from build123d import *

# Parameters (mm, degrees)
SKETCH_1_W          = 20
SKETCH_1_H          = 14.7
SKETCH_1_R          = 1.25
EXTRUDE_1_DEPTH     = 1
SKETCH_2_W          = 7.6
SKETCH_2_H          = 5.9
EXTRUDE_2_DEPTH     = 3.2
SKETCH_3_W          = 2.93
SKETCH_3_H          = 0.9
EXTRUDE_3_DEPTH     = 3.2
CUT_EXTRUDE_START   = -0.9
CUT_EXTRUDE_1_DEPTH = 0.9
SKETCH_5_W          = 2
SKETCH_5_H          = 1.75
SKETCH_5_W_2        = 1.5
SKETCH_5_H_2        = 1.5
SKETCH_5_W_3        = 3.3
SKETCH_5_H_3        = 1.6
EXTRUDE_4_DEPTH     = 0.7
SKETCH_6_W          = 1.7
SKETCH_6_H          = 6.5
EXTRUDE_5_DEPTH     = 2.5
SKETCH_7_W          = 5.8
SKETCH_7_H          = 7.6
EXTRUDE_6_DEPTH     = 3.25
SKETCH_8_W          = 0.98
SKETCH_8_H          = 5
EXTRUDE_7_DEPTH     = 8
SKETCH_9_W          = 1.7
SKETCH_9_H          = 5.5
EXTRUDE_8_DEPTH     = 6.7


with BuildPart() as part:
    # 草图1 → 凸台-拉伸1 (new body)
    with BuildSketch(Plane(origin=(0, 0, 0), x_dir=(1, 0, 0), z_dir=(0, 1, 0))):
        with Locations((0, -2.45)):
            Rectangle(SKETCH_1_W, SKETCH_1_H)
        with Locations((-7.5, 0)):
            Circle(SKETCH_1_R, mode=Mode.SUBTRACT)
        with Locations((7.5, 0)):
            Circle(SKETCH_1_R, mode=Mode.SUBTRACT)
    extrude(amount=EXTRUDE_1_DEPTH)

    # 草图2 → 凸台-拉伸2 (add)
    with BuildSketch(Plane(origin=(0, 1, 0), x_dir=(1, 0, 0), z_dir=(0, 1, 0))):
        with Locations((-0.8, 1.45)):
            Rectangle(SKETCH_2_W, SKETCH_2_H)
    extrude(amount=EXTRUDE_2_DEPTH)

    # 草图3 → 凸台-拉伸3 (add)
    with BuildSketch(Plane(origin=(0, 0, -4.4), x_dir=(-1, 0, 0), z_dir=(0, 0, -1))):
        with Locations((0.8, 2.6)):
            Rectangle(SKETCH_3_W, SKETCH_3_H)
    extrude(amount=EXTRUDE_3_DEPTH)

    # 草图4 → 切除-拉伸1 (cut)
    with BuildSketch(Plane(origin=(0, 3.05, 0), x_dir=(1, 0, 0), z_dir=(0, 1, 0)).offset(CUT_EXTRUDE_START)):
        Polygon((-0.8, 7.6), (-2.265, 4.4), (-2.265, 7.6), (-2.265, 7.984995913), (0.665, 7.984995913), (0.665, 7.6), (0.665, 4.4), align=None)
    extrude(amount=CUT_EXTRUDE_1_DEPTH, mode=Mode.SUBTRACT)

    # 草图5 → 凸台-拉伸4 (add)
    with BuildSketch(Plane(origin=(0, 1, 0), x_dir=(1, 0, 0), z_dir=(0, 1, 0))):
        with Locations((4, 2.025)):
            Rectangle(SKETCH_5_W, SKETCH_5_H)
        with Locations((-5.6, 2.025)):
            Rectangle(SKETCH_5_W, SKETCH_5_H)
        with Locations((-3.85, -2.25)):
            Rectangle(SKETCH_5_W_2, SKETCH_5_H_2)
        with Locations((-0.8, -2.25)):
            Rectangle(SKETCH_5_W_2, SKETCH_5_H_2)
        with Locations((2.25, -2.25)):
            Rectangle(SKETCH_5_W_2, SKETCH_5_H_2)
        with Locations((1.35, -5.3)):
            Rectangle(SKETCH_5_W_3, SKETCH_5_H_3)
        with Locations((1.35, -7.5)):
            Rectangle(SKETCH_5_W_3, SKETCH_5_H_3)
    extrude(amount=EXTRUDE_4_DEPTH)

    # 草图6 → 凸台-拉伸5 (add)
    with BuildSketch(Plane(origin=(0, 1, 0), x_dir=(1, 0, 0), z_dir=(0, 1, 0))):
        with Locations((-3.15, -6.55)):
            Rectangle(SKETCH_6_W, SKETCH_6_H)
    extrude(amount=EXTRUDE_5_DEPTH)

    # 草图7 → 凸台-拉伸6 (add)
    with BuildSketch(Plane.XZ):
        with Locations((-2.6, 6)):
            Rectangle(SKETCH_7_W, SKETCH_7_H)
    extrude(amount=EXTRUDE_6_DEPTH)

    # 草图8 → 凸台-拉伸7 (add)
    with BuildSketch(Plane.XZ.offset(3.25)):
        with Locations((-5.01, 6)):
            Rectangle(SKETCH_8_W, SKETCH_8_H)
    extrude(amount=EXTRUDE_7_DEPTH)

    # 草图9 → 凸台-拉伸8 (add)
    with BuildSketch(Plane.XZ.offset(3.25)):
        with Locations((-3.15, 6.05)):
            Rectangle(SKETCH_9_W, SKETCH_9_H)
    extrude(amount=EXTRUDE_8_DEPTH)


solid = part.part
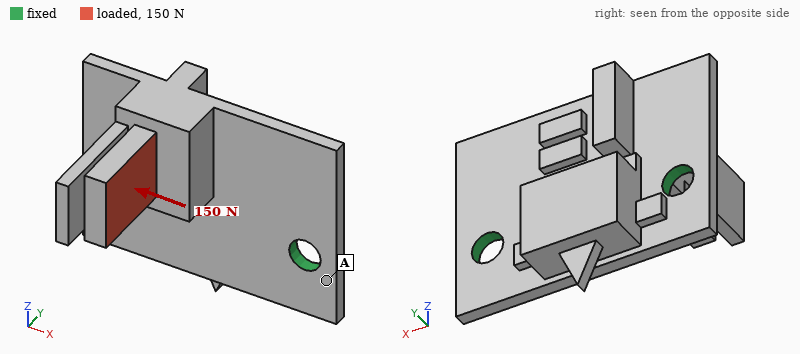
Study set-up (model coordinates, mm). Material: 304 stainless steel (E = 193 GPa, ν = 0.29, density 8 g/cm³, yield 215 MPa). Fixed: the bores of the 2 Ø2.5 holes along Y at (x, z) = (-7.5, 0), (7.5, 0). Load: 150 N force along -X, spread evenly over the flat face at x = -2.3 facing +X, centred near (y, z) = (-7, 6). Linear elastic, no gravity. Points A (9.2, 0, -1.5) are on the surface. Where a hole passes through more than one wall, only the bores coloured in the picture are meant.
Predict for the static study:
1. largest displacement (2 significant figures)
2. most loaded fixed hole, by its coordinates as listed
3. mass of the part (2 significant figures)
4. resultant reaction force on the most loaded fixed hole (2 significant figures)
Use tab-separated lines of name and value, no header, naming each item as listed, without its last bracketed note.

largest displacement	36 µm
most loaded fixed hole, by its coordinates as listed	(-7.5, 0)
mass of the part	5.8 g
resultant reaction force on the most loaded fixed hole	160 N
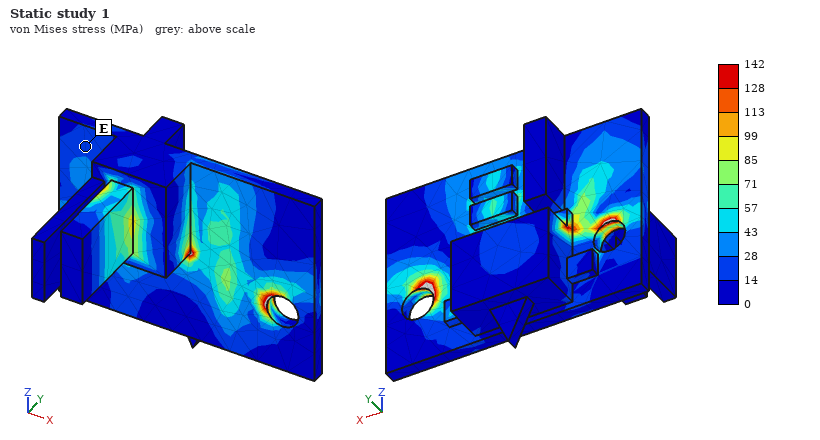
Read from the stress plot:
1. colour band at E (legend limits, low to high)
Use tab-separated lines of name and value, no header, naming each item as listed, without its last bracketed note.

colour band at E	14 to 28 MPa
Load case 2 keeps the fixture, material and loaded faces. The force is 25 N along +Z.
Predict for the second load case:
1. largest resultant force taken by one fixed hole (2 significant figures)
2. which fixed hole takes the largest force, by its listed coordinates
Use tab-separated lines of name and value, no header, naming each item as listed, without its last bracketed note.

largest resultant force taken by one fixed hole	16 N
which fixed hole takes the largest force, by its listed coordinates	(-7.5, 0)
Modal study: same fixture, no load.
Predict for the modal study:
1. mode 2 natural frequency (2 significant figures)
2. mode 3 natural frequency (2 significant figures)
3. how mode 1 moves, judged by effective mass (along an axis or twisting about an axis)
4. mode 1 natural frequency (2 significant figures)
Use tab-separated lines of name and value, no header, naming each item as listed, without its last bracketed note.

mode 2 natural frequency	9900 Hz
mode 3 natural frequency	15 kHz
how mode 1 moves, judged by effective mass	along Y
mode 1 natural frequency	5000 Hz
